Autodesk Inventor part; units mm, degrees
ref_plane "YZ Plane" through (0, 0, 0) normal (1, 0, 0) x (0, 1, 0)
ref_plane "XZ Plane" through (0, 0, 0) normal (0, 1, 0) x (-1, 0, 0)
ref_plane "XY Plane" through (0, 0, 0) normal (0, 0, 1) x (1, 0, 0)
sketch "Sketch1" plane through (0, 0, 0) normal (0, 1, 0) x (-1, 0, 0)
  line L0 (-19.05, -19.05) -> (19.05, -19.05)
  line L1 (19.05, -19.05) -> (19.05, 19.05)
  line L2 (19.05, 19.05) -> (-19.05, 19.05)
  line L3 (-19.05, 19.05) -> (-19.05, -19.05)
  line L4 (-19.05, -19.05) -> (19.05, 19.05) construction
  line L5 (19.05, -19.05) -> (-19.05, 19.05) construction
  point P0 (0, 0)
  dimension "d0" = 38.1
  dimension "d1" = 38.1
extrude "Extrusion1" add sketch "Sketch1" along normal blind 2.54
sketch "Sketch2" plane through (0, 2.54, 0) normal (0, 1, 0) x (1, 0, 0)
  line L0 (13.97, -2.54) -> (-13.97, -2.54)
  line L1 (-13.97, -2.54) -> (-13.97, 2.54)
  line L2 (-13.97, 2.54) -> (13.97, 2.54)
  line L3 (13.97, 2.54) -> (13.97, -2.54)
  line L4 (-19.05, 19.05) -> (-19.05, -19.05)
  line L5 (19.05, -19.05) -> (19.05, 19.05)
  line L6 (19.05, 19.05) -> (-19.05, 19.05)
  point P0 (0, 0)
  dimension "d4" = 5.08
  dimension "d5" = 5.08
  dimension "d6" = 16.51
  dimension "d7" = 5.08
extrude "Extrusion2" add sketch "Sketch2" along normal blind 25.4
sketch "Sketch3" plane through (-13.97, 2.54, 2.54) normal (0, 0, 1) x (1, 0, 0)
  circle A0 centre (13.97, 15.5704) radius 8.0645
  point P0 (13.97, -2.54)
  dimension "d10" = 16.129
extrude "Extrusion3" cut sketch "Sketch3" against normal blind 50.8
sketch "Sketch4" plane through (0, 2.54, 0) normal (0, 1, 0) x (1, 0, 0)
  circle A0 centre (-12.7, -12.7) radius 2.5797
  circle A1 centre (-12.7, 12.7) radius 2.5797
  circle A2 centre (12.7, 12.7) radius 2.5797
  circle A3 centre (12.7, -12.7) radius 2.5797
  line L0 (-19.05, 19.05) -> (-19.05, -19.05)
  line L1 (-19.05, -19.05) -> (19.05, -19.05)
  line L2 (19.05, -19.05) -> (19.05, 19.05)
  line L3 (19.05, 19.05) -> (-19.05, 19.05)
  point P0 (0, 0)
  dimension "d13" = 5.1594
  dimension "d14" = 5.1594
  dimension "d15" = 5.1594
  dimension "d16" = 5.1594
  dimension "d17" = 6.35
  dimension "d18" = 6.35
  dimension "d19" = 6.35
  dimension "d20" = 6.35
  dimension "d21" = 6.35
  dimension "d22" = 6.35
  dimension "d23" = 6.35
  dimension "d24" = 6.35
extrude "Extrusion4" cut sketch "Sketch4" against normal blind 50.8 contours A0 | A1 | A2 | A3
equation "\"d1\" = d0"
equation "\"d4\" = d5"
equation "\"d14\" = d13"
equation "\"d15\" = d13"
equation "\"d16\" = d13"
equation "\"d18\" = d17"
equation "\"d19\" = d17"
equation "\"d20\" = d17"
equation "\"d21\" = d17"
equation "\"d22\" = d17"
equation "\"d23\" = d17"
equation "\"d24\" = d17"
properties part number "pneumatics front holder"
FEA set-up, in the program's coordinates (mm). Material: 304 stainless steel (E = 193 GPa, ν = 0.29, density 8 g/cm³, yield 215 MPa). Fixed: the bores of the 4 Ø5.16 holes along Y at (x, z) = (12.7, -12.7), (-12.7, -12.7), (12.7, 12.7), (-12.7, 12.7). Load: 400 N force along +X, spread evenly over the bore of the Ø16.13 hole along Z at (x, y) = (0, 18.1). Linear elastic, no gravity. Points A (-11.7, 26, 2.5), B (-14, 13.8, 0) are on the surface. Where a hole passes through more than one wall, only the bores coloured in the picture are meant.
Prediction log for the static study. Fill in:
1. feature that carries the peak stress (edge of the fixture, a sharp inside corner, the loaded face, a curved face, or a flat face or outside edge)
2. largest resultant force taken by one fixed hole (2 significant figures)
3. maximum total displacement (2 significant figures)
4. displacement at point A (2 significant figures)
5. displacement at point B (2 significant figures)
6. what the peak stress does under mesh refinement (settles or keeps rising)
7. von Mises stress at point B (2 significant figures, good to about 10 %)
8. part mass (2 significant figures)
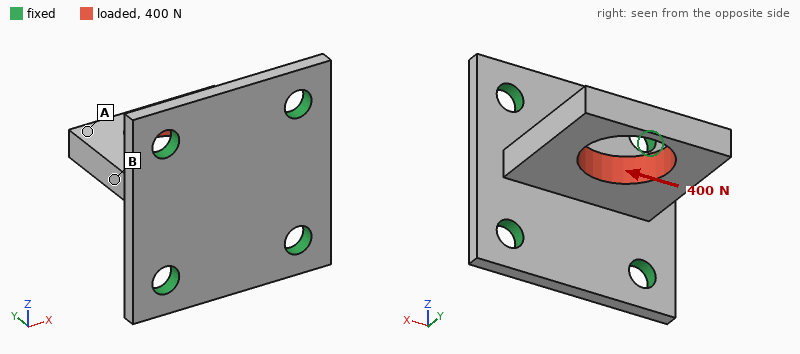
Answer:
edge of the fixture
170 N
14 µm
12 µm
6.8 µm
keeps rising
16 MPa
48 g
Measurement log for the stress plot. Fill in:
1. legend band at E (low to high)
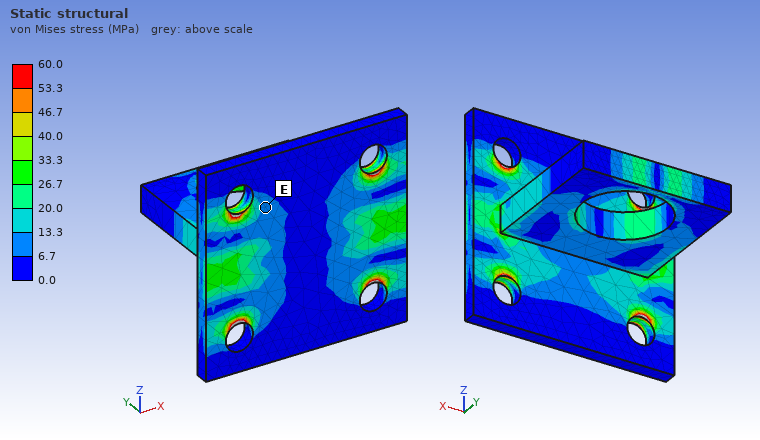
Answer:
6.7 to 13.3 MPa
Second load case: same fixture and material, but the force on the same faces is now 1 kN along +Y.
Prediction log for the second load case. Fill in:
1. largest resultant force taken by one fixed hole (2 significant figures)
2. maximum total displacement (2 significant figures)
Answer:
260 N
9.9 µm
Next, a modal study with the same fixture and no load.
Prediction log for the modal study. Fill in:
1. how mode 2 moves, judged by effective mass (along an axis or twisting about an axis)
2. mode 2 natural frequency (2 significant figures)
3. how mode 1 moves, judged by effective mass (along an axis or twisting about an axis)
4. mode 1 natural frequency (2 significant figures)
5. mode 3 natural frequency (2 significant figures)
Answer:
along X
8000 Hz
along Z
4600 Hz
9100 Hz
